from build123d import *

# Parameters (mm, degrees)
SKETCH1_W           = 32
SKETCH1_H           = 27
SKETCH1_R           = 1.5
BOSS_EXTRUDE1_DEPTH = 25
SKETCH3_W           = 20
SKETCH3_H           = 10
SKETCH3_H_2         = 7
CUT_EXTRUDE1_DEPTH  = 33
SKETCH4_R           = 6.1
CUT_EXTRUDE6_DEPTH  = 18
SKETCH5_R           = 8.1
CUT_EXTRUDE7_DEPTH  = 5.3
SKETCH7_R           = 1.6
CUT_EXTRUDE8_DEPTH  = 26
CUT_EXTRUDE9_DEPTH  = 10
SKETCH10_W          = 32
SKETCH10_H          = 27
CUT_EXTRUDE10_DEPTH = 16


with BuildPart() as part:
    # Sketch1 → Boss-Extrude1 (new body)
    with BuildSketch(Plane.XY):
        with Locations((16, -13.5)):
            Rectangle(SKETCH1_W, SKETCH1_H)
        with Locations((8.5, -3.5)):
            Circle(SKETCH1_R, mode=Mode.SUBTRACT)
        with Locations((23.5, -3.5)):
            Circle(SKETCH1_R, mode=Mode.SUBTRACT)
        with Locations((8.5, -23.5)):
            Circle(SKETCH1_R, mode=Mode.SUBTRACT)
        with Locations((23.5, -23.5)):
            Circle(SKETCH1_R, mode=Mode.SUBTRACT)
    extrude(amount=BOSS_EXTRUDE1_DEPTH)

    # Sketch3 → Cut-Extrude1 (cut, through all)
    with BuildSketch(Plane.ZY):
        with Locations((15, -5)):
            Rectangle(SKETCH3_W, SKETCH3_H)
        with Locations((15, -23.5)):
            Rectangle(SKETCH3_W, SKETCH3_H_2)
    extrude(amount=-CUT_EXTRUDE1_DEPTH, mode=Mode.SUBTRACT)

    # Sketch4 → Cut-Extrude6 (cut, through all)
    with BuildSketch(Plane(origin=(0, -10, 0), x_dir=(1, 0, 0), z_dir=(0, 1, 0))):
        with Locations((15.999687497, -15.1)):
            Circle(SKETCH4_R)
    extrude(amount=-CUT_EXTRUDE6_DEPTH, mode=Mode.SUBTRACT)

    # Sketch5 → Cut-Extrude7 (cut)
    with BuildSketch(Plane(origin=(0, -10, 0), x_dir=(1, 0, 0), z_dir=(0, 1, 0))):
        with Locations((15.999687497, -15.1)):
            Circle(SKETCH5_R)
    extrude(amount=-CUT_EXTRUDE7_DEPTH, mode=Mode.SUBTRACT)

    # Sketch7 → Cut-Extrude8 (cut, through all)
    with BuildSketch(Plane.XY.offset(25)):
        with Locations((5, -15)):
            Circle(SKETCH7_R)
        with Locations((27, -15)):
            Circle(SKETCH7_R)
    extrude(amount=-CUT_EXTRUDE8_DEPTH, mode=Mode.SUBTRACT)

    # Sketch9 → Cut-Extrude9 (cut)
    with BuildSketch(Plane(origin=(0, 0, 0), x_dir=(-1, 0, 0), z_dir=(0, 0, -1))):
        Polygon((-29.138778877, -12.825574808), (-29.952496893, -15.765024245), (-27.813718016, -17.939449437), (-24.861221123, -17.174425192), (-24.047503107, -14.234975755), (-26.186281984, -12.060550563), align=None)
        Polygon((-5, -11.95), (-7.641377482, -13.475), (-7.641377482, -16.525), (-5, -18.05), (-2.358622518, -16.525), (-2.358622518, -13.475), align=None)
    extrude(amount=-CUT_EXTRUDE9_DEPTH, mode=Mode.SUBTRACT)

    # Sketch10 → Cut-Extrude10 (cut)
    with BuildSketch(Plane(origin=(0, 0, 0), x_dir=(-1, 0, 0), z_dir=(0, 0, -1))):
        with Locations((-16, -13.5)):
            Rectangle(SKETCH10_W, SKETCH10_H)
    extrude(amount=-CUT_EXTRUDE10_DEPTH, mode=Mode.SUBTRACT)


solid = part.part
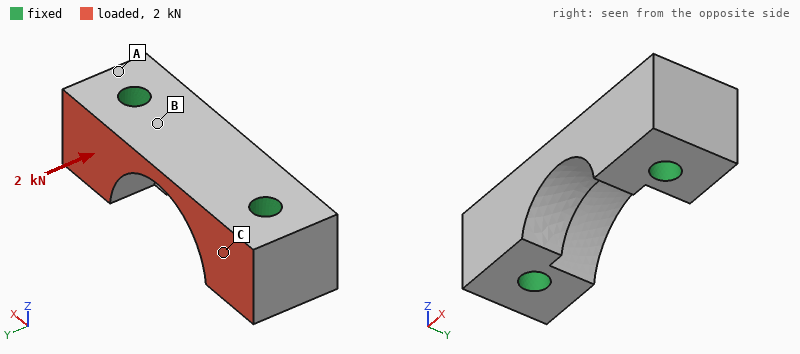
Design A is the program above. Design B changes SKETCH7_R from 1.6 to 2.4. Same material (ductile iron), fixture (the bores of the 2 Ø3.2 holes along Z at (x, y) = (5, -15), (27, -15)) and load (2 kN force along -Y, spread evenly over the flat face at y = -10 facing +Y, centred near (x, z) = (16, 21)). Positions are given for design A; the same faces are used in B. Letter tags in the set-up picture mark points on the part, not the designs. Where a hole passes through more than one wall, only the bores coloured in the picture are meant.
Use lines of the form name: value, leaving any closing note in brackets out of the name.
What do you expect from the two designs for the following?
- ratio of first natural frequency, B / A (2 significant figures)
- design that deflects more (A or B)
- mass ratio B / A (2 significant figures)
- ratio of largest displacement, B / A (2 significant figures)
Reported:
ratio of first natural frequency, B / A: 1.2
design that deflects more: A
mass ratio B / A: 0.91
ratio of largest displacement, B / A: 0.82
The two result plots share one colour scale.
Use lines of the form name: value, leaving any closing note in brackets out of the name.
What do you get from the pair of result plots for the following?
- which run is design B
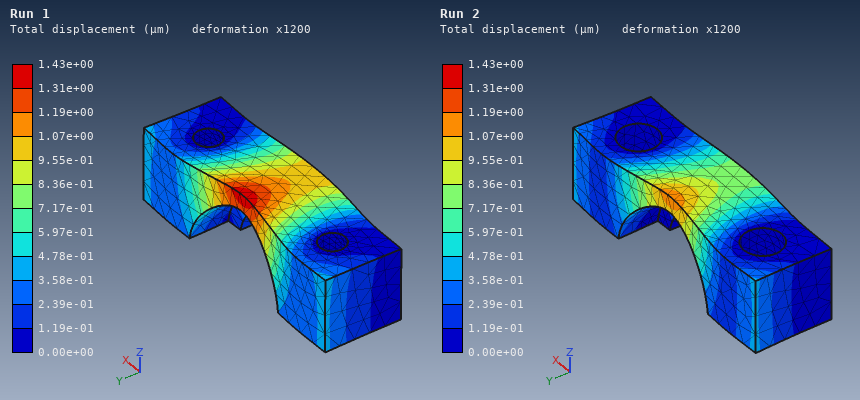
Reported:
which run is design B: Run 2
